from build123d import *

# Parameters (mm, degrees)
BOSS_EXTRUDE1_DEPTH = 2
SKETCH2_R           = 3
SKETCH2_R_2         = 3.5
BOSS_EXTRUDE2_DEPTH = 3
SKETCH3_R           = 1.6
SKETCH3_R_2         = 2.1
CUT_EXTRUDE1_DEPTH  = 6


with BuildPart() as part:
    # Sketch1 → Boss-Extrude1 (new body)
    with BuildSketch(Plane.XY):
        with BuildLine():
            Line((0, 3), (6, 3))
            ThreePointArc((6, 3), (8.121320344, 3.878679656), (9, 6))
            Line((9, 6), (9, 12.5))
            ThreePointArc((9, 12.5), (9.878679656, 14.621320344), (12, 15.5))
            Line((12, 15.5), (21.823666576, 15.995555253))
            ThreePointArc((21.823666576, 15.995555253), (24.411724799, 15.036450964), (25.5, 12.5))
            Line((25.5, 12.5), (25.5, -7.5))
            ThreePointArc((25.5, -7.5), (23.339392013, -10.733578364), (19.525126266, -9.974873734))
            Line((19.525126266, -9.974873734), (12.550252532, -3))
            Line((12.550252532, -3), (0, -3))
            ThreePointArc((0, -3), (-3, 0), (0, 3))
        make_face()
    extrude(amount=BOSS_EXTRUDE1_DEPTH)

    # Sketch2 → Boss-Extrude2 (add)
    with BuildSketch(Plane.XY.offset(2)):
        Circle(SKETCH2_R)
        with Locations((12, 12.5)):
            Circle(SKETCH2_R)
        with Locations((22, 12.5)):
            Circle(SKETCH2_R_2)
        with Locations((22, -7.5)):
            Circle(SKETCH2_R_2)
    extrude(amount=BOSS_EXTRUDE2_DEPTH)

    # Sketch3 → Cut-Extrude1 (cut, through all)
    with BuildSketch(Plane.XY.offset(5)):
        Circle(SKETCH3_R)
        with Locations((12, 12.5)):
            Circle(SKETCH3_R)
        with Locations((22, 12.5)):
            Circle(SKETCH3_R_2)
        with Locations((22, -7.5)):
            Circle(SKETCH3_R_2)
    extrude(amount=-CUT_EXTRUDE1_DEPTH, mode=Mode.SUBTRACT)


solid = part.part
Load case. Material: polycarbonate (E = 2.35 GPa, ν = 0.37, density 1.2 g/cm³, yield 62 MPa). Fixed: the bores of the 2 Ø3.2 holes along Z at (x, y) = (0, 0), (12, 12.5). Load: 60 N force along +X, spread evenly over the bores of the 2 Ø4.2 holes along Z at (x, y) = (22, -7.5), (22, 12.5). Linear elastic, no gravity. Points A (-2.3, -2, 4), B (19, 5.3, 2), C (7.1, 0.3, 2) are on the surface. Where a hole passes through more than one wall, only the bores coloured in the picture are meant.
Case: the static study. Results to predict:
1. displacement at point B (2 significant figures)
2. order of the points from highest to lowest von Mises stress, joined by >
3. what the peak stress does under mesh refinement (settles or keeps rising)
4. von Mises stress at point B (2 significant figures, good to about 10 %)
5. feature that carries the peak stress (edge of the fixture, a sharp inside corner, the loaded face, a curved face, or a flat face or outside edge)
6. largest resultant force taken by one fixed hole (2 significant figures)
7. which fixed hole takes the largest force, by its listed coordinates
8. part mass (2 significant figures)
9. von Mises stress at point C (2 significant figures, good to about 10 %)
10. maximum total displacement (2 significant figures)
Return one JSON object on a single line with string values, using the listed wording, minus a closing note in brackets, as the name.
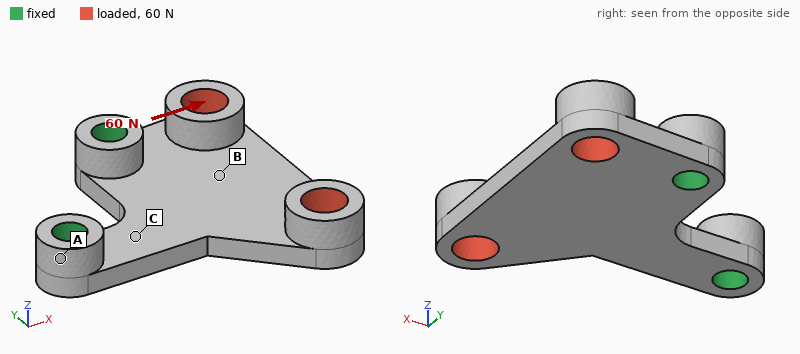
{"displacement at point B": "0.097 mm", "order of the points from highest to lowest von Mises stress, joined by >": "C > B > A", "what the peak stress does under mesh refinement": "keeps rising", "von Mises stress at point B": "4.0 MPa", "feature that carries the peak stress": "a sharp inside corner", "largest resultant force taken by one fixed hole": "41 N", "which fixed hole takes the largest force, by its listed coordinates": "(0, 0)", "part mass": "1.3 g", "von Mises stress at point C": "5.8 MPa", "maximum total displacement": "0.40 mm"}
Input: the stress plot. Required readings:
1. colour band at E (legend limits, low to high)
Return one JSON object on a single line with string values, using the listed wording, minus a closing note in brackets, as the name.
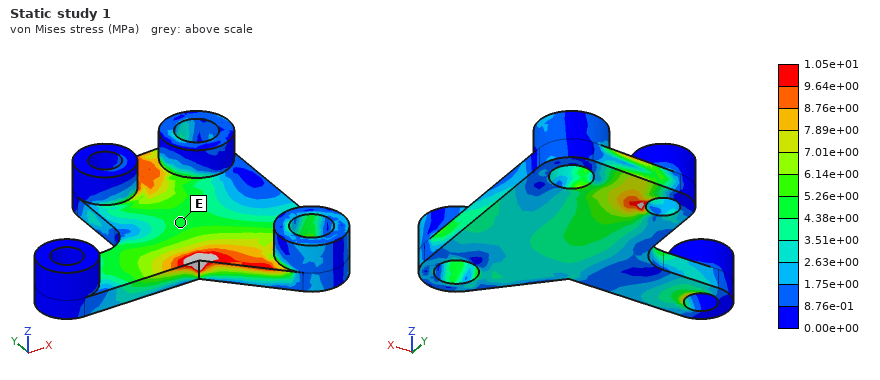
{"colour band at E": "4.38e+00 to 5.26e+00 MPa"}
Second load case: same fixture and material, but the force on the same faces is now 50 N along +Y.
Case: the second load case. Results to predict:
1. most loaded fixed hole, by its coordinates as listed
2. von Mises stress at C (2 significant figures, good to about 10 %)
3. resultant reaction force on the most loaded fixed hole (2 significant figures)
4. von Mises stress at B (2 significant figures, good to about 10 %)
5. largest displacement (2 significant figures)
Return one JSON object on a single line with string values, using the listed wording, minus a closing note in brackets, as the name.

{"most loaded fixed hole, by its coordinates as listed": "(12, 12.5)", "von Mises stress at C": "2.5 MPa", "resultant reaction force on the most loaded fixed hole": "59 N", "von Mises stress at B": "4.9 MPa", "largest displacement": "0.45 mm"}
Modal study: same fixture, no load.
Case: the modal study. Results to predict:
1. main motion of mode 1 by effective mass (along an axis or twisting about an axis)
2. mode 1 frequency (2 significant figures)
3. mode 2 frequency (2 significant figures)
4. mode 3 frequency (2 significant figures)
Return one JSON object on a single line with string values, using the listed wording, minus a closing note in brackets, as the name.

{"main motion of mode 1 by effective mass": "along Z", "mode 1 frequency": "1000 Hz", "mode 2 frequency": "2800 Hz", "mode 3 frequency": "4900 Hz"}
